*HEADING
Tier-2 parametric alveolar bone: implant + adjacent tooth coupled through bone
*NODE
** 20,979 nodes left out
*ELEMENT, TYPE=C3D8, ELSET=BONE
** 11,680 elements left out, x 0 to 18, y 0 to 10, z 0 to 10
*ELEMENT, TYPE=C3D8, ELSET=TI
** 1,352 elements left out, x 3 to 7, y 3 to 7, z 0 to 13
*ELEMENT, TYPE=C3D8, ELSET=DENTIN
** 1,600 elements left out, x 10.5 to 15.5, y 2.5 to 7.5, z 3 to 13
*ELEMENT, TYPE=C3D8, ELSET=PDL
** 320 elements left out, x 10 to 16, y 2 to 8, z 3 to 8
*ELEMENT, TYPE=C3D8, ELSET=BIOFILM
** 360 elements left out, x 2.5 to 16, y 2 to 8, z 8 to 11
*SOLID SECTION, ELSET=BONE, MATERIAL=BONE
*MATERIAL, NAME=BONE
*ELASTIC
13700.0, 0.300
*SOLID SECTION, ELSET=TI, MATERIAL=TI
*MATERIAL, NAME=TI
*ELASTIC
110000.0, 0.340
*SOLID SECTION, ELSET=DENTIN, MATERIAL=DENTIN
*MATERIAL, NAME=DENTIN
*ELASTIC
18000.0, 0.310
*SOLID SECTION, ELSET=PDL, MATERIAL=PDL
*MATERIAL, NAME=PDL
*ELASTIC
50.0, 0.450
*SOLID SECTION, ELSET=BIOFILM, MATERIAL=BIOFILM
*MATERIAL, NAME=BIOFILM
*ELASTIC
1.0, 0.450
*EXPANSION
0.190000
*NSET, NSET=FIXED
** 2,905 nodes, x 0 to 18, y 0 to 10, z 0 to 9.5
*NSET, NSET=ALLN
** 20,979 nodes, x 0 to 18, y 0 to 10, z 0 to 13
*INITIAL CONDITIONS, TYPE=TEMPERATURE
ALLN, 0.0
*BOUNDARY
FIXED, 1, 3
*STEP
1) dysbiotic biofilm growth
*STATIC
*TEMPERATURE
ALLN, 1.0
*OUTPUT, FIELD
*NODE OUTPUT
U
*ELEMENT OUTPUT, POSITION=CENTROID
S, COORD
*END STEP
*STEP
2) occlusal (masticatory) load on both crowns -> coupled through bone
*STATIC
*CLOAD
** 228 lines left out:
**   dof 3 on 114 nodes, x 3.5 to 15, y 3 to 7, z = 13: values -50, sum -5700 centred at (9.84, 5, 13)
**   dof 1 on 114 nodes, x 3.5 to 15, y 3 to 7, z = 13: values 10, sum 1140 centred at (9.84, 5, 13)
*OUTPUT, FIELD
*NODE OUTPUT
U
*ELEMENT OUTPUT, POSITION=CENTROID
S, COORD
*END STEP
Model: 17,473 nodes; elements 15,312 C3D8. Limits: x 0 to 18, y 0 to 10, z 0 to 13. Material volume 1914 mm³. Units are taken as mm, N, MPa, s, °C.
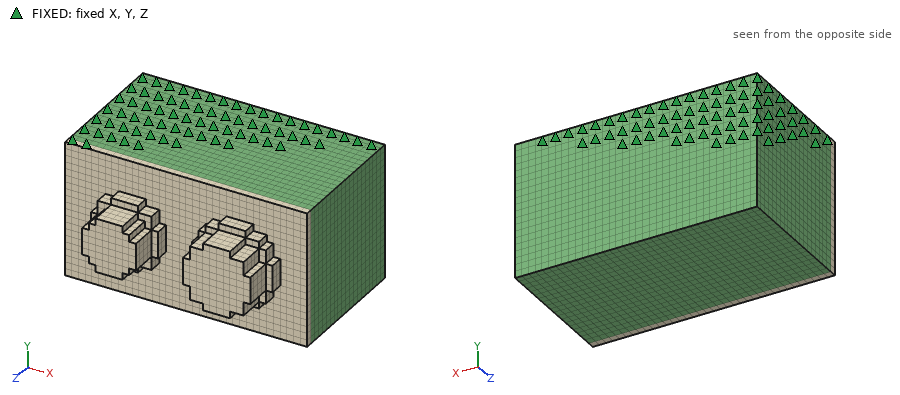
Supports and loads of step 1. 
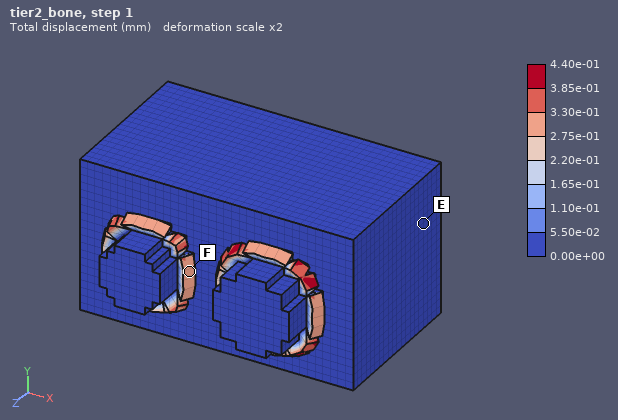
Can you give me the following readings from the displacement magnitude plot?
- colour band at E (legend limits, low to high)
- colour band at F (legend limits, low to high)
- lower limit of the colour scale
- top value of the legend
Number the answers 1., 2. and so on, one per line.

1. 0.00e+00 to 5.50e-02 mm
2. 2.75e-01 to 3.30e-01 mm
3. 0.00e+00 mm
4. 4.40e-01 mm
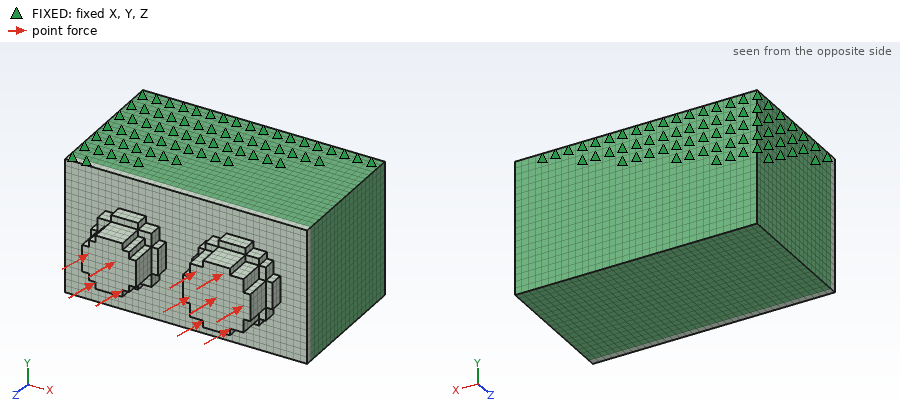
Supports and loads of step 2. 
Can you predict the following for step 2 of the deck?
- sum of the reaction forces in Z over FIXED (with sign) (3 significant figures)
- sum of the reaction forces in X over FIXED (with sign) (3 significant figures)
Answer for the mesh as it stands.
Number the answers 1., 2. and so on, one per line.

1. 5700 N
2. -1140 N
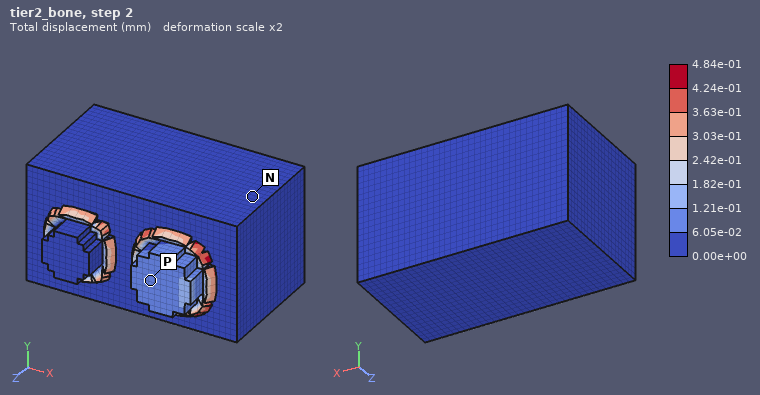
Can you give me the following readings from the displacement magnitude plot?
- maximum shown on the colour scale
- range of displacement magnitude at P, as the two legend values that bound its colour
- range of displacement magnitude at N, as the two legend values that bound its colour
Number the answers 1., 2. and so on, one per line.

1. 4.84e-01 mm
2. 6.05e-02 to 1.21e-01 mm
3. 0.00e+00 to 6.05e-02 mm
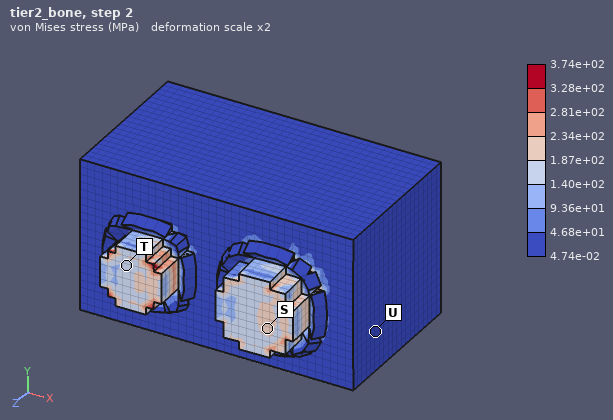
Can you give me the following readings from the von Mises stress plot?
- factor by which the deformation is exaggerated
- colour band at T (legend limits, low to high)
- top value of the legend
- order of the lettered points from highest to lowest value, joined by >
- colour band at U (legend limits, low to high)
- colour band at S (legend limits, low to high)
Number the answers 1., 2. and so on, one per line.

1. 2
2. 1.40e+02 to 1.87e+02 MPa
3. 3.74e+02 MPa
4. S > T > U
5. 4.74e-02 to 4.68e+01 MPa
6. 1.87e+02 to 2.34e+02 MPa
